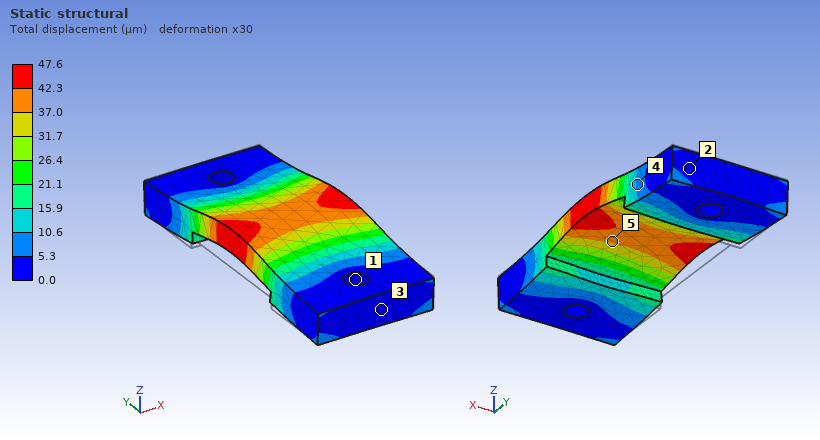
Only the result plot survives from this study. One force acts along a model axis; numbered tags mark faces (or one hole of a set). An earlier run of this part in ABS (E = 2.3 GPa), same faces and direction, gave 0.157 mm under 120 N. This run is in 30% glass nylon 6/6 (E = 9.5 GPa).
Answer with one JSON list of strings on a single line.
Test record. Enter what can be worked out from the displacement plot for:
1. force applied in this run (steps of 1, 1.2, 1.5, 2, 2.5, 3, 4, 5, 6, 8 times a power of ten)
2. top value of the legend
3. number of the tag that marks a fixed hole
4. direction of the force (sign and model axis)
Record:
["150 N", "47.6 µm", "1", "+Z"]
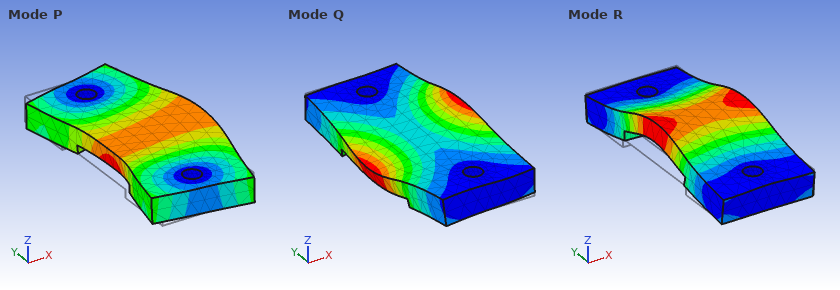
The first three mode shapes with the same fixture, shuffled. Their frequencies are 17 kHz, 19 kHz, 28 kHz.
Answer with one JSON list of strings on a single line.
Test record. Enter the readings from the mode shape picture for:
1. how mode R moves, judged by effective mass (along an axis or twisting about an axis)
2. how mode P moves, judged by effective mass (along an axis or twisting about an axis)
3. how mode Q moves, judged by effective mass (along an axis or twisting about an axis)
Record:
["along Z", "along X", "twisting about Y"]
